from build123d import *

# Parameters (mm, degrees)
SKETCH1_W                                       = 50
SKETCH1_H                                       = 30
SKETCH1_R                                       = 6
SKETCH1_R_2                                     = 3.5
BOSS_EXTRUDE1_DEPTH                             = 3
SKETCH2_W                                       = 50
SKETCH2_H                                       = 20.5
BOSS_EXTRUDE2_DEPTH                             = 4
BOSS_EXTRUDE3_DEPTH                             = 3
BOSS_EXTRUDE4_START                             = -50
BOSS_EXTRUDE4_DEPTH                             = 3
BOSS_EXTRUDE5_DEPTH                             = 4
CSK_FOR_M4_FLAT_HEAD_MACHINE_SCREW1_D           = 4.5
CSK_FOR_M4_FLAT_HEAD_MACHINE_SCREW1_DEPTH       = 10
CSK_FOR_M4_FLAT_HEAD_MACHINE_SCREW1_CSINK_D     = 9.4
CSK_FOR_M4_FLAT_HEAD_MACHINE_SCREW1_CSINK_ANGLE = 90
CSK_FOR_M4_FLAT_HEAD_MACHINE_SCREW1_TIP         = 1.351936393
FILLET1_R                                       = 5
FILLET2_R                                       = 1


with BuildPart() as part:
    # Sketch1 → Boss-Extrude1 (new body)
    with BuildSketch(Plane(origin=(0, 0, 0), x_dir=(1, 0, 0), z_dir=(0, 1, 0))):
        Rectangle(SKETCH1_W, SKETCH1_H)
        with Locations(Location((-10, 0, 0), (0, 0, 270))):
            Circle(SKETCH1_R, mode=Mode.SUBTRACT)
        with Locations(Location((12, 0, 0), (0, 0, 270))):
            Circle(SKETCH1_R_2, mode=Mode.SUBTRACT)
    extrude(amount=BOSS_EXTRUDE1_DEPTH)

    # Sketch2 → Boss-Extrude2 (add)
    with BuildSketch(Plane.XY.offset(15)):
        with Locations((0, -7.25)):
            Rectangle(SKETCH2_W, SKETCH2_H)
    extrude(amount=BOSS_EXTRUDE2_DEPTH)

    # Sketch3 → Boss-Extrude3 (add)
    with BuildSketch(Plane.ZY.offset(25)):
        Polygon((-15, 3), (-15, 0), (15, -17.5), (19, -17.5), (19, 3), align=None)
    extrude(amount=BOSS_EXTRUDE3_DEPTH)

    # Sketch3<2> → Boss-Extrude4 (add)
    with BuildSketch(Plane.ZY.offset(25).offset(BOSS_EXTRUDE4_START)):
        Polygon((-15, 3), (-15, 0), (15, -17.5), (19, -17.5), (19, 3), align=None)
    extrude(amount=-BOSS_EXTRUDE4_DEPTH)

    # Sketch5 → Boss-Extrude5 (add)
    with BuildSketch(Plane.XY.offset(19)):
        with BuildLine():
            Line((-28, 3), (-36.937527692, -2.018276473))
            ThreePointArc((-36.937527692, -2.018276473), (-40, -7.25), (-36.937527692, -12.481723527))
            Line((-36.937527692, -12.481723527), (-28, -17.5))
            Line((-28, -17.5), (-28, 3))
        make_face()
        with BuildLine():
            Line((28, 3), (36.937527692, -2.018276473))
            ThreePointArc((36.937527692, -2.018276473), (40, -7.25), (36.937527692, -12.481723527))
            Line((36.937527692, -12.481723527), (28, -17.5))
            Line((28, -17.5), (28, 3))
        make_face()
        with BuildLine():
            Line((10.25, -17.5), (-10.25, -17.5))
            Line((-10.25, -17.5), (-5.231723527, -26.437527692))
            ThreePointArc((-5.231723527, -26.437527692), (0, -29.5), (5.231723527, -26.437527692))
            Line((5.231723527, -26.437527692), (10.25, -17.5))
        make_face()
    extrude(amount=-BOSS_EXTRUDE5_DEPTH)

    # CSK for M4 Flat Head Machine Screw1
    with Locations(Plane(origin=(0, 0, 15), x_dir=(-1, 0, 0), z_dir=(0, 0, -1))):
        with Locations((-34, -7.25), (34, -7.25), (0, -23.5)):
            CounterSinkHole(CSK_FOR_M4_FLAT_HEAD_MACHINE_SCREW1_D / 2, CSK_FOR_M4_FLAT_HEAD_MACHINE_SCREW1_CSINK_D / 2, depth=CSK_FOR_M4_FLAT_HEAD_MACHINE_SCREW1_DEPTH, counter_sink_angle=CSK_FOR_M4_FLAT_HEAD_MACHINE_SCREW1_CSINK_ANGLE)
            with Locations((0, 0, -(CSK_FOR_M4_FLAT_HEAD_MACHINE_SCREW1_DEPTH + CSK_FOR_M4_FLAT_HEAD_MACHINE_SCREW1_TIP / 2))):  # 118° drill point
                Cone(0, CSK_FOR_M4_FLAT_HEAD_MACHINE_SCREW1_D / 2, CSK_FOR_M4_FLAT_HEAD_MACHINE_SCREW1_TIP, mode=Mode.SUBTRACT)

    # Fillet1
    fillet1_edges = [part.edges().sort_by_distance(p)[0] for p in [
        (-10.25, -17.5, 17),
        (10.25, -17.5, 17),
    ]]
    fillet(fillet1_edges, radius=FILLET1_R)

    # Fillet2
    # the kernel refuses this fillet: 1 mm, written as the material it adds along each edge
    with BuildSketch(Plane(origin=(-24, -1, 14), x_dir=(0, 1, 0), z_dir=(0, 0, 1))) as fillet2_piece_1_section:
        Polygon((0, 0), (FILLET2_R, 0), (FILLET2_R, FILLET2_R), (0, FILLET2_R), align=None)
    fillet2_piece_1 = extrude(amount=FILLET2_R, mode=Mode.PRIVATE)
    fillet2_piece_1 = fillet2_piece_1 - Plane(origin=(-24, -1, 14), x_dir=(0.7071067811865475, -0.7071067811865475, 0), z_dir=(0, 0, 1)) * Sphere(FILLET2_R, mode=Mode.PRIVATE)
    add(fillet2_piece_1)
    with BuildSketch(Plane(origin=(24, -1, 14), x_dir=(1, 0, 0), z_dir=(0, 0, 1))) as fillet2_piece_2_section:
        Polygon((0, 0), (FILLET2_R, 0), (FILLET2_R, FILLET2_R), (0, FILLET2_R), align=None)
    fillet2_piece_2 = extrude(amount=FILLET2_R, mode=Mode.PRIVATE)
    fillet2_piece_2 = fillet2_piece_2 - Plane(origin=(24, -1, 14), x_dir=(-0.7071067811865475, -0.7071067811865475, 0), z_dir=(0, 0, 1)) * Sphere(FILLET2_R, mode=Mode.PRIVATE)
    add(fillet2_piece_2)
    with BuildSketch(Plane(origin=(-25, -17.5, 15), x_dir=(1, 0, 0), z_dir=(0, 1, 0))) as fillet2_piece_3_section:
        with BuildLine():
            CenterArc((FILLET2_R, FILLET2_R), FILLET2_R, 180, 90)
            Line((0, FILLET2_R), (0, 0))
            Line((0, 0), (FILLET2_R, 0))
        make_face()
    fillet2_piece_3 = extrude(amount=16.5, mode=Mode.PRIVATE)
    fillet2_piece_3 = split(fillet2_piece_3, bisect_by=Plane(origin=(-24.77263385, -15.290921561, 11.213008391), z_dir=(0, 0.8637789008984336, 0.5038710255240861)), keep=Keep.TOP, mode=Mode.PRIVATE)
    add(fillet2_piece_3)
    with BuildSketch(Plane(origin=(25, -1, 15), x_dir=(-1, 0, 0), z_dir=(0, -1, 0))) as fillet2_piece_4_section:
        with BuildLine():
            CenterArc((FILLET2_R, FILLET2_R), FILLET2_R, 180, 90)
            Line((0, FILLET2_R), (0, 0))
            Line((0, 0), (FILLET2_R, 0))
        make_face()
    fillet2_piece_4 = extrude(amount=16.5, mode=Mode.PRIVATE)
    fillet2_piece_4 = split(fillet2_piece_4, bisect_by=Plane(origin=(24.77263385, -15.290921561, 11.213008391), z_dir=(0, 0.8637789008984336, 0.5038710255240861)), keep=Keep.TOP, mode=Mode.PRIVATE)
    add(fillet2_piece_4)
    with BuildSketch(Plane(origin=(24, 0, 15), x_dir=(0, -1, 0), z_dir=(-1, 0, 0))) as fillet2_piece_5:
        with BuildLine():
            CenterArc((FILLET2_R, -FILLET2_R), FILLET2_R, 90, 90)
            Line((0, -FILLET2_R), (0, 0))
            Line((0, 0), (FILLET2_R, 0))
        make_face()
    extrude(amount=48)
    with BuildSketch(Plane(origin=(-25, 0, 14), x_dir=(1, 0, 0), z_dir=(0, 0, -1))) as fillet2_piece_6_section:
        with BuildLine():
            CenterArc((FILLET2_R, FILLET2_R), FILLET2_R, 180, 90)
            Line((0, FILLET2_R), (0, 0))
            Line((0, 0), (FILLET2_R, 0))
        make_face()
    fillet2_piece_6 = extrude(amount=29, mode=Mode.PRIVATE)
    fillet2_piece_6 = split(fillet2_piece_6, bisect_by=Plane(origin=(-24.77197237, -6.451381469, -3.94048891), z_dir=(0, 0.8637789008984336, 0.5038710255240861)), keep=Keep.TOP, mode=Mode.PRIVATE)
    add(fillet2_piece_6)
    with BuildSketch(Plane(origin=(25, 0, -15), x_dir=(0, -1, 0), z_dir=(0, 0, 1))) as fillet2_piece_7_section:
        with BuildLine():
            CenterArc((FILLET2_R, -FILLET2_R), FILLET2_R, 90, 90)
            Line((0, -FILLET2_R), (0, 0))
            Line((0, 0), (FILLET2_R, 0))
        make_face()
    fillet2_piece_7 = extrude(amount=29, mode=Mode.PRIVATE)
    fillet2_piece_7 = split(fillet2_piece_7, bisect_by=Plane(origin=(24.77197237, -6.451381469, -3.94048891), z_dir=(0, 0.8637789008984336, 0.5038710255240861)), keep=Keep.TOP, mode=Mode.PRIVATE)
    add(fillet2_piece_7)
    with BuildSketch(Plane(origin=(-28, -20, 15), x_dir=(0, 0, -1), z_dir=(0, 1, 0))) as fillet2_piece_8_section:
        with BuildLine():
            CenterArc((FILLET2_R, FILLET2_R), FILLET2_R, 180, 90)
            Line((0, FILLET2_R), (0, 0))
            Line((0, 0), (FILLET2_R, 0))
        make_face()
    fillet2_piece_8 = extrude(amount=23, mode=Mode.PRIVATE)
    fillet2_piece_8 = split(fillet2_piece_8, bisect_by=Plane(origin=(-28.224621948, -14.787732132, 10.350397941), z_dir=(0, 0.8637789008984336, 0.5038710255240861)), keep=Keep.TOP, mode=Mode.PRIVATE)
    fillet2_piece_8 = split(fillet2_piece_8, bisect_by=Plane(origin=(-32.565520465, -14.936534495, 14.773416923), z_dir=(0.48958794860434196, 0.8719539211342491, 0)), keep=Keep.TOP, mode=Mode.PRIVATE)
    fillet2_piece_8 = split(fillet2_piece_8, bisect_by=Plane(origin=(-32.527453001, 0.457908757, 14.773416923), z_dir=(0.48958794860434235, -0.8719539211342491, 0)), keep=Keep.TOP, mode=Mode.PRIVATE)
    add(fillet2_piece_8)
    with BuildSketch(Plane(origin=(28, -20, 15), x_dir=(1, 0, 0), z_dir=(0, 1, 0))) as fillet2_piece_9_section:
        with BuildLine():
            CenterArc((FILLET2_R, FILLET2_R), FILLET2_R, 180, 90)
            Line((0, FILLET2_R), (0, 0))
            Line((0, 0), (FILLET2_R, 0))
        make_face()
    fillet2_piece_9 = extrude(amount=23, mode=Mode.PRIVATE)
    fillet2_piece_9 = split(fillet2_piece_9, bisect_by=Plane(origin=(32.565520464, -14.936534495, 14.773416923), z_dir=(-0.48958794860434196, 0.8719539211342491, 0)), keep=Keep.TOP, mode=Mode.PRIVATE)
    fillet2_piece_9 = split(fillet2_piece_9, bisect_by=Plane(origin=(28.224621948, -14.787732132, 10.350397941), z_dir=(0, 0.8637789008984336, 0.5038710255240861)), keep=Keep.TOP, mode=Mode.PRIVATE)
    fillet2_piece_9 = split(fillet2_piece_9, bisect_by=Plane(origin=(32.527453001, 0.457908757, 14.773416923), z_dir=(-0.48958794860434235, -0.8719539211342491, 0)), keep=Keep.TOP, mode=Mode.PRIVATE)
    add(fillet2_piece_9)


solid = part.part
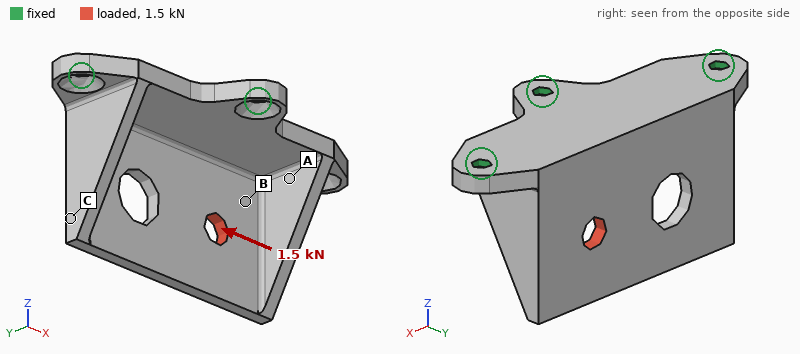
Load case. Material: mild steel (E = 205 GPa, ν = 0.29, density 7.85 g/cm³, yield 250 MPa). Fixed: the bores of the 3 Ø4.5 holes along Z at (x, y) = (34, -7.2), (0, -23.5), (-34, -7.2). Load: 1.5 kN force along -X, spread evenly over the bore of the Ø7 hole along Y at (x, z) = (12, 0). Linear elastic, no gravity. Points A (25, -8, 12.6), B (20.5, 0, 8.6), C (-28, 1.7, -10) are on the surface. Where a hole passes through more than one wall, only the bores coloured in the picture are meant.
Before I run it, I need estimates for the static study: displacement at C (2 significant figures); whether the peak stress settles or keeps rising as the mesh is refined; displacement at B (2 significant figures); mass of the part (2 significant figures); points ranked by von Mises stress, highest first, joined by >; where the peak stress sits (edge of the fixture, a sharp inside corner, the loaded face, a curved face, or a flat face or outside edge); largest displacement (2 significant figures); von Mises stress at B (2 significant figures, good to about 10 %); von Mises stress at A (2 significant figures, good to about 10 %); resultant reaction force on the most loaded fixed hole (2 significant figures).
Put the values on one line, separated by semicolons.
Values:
22 µm; keeps rising; 6.9 µm; 97 g; B > A > C; edge of the fixture; 25 µm; 29 MPa; 19 MPa; 810 N
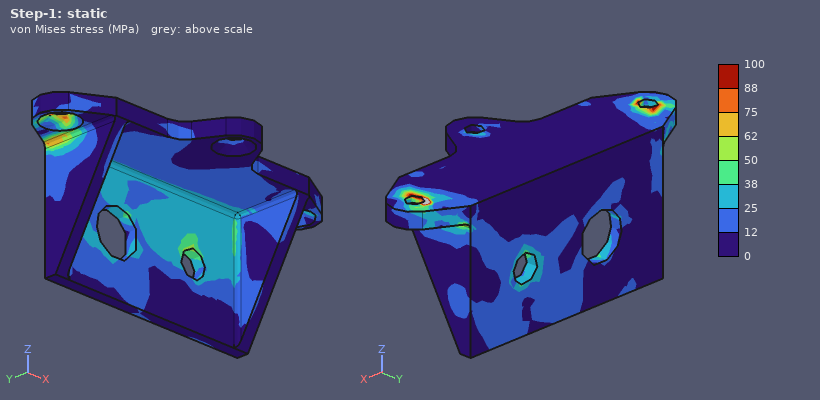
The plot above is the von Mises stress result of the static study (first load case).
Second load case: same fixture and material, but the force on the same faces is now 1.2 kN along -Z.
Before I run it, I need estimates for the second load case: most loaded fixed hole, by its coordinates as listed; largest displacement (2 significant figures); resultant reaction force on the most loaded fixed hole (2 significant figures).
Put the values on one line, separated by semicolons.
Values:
(34, -7.2); 71 µm; 1.1 kN
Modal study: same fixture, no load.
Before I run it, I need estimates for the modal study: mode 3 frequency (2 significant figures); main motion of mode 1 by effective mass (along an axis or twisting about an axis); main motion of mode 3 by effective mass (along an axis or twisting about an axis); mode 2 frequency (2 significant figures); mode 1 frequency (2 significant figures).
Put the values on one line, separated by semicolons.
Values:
7100 Hz; along Y; along Z; 4700 Hz; 2700 Hz
